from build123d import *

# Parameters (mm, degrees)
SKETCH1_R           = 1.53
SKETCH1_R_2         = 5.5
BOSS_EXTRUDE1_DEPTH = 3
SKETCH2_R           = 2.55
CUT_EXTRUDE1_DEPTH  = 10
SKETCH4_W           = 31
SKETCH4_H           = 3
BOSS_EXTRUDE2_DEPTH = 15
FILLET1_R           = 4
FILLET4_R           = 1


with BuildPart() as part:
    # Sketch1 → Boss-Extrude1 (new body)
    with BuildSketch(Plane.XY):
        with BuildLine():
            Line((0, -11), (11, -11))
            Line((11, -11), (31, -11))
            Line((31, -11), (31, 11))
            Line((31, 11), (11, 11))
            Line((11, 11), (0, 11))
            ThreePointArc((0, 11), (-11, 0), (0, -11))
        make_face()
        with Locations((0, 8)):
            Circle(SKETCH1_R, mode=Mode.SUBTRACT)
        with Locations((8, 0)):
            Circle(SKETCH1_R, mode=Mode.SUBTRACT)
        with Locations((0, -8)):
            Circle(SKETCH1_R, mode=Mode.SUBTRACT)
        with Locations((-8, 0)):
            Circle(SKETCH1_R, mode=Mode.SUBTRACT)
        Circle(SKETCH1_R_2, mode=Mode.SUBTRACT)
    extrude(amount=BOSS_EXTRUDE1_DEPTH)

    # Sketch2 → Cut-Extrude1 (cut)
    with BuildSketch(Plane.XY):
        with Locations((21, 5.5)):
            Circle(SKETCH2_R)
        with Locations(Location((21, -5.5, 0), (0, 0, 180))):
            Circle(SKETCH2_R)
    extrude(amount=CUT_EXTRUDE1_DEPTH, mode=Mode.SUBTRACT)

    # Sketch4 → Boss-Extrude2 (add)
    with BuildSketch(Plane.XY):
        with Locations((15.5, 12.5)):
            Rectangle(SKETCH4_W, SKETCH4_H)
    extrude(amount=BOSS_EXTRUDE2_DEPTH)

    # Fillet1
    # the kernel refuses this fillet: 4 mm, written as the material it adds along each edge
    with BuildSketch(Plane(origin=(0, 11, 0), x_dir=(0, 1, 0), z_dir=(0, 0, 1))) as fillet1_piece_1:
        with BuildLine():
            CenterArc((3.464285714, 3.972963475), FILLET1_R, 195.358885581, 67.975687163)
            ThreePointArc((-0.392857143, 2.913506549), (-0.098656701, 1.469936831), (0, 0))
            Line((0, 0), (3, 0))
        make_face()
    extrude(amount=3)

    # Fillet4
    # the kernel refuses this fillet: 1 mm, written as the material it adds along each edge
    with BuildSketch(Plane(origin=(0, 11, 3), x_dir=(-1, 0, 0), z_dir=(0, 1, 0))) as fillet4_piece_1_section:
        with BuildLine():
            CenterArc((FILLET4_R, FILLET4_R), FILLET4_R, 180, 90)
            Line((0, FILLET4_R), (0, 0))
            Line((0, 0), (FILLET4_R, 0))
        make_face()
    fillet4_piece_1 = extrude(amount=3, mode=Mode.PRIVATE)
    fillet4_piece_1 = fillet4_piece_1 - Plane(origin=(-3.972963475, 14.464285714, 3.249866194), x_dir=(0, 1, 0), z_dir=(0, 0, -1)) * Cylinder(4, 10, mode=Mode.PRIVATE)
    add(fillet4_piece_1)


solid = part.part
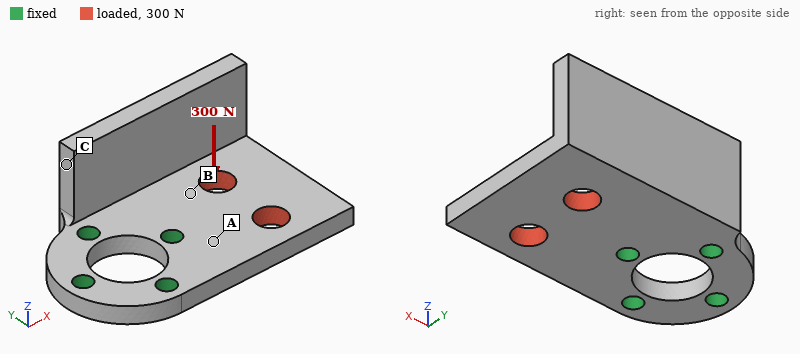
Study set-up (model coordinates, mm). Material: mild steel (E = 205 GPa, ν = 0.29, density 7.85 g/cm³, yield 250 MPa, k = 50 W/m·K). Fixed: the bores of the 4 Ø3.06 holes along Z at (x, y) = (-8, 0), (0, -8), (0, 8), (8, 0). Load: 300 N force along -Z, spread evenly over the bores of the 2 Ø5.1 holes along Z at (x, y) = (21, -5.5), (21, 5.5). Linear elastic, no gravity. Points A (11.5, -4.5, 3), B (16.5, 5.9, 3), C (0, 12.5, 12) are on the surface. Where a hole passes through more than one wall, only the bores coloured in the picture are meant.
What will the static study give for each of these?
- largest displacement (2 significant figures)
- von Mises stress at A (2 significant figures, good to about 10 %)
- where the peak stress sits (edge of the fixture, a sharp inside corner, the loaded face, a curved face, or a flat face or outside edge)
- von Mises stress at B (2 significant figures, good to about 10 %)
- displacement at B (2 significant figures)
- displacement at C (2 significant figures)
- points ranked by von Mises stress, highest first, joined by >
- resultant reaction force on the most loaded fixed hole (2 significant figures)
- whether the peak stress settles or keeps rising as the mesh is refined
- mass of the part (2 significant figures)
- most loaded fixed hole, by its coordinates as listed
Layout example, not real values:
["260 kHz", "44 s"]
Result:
["36 µm", "53 MPa", "edge of the fixture", "29 MPa", "10 µm", "8.3 µm", "A > B > C", "420 N", "keeps rising", "28 g", "(8, 0)"]
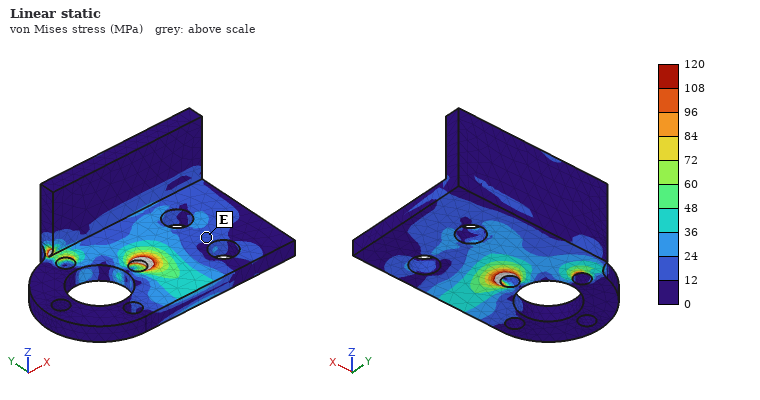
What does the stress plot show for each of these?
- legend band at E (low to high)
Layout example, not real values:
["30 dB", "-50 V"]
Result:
["12 to 24 MPa"]
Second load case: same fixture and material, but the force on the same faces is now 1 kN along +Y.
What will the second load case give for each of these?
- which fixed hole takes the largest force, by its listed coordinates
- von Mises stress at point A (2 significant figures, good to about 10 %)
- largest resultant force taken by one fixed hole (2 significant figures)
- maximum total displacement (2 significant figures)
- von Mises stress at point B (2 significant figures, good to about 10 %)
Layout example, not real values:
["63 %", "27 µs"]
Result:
["(8, 0)", "34 MPa", "1.1 kN", "9.5 µm", "40 MPa"]
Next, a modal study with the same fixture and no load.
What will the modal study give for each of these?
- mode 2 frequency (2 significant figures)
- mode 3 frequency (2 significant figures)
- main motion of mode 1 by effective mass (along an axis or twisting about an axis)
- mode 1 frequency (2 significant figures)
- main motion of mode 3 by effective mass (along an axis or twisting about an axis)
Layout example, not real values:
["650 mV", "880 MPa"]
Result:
["6200 Hz", "10 kHz", "along Z", "3700 Hz", "along Y"]
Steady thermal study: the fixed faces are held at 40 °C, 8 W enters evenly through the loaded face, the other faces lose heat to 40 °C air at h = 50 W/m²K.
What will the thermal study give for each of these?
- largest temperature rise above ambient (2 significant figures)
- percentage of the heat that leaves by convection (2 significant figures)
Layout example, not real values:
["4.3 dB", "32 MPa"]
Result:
["31 K", "22 %"]
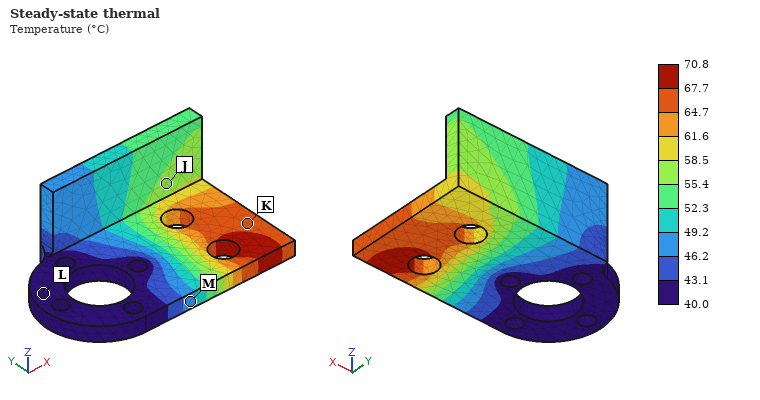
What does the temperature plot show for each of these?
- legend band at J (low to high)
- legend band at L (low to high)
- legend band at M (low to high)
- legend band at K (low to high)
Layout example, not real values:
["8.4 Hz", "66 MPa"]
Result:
["55.4 to 58.5 °C", "40.0 to 43.1 °C", "46.2 to 49.2 °C", "64.7 to 67.7 °C"]
